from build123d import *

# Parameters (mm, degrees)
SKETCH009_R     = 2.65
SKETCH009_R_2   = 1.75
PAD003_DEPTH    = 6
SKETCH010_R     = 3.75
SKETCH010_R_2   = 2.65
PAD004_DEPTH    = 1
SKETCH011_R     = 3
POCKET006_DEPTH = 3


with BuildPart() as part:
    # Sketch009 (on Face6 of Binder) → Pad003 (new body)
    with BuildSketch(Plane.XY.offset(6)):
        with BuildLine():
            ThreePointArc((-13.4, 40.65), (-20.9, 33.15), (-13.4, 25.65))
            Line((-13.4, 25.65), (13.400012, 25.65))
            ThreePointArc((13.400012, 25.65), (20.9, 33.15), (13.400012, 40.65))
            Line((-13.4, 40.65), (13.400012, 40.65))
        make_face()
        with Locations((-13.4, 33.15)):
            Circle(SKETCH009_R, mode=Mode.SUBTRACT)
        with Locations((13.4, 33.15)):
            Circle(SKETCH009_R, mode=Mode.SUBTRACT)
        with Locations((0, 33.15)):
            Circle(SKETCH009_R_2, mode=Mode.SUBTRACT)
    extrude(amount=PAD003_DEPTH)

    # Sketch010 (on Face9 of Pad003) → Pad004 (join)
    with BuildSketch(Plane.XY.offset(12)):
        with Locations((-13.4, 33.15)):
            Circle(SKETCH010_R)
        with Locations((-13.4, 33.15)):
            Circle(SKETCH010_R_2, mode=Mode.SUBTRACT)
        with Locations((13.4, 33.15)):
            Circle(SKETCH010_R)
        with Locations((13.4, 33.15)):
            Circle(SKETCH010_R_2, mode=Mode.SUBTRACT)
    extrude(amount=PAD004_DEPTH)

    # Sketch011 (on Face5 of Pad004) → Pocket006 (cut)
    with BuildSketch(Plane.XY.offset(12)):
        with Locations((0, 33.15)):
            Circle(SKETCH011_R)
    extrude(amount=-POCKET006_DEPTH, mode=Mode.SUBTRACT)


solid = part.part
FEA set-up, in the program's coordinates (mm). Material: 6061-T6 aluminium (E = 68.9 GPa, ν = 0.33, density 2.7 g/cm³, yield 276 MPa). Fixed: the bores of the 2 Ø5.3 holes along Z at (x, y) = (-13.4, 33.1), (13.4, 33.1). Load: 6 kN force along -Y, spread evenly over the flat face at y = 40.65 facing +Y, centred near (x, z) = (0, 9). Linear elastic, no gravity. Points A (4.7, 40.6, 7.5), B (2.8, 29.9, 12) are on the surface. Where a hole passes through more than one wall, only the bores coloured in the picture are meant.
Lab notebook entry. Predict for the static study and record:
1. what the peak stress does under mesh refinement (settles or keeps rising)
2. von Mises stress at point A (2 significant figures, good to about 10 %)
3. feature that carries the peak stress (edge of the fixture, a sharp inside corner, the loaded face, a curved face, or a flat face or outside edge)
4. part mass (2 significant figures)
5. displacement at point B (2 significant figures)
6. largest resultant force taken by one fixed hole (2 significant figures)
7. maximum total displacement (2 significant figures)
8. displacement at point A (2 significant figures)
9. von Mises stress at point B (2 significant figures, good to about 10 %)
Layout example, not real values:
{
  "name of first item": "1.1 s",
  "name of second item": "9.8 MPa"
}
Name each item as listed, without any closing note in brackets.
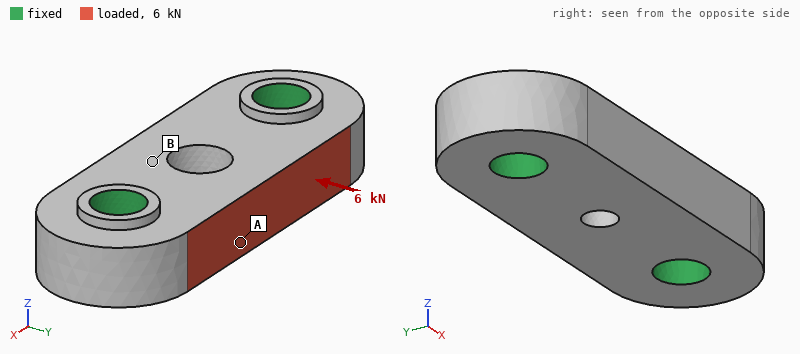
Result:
{
  "what the peak stress does under mesh refinement": "keeps rising",
  "von Mises stress at point A": "44 MPa",
  "feature that carries the peak stress": "edge of the fixture",
  "part mass": "8.5 g",
  "displacement at point B": "9.4 µm",
  "largest resultant force taken by one fixed hole": "3.1 kN",
  "maximum total displacement": "16 µm",
  "displacement at point A": "13 µm",
  "von Mises stress at point B": "17 MPa"
}
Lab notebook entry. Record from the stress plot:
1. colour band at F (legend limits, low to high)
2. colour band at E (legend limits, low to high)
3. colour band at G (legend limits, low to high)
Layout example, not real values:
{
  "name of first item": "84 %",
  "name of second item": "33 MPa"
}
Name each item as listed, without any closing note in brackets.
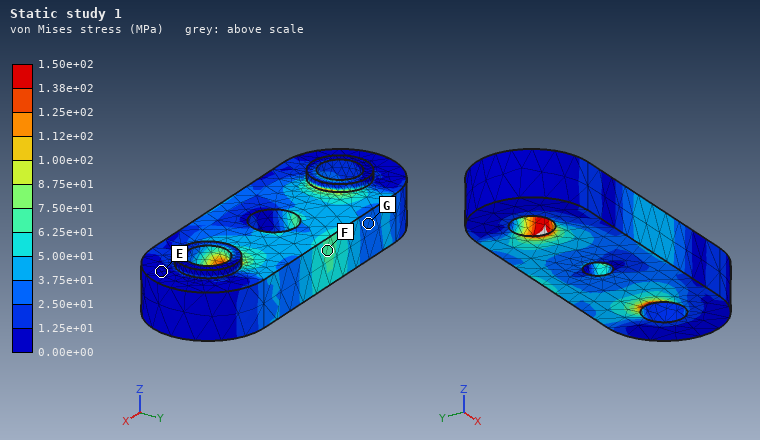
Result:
{
  "colour band at F": "6.25e+01 to 7.50e+01 MPa",
  "colour band at E": "0.00e+00 to 1.25e+01 MPa",
  "colour band at G": "2.50e+01 to 3.75e+01 MPa"
}
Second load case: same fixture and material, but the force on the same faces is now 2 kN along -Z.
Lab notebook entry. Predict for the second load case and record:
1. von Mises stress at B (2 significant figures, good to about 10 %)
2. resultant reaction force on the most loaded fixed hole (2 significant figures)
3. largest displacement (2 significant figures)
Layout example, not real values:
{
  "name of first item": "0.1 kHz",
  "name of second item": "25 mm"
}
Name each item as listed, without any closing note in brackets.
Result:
{
  "von Mises stress at B": "14 MPa",
  "resultant reaction force on the most loaded fixed hole": "1.0 kN",
  "largest displacement": "27 µm"
}
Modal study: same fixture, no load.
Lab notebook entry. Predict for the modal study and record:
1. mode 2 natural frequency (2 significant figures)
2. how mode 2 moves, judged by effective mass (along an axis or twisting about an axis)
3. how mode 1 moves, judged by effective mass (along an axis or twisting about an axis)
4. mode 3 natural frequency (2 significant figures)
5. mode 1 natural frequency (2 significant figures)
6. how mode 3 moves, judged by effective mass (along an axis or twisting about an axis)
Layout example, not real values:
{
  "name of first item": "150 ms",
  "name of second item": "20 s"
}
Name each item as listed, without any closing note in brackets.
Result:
{
  "mode 2 natural frequency": "44 kHz",
  "how mode 2 moves, judged by effective mass": "twisting about X",
  "how mode 1 moves, judged by effective mass": "along Z",
  "mode 3 natural frequency": "51 kHz",
  "mode 1 natural frequency": "40 kHz",
  "how mode 3 moves, judged by effective mass": "along Y"
}
